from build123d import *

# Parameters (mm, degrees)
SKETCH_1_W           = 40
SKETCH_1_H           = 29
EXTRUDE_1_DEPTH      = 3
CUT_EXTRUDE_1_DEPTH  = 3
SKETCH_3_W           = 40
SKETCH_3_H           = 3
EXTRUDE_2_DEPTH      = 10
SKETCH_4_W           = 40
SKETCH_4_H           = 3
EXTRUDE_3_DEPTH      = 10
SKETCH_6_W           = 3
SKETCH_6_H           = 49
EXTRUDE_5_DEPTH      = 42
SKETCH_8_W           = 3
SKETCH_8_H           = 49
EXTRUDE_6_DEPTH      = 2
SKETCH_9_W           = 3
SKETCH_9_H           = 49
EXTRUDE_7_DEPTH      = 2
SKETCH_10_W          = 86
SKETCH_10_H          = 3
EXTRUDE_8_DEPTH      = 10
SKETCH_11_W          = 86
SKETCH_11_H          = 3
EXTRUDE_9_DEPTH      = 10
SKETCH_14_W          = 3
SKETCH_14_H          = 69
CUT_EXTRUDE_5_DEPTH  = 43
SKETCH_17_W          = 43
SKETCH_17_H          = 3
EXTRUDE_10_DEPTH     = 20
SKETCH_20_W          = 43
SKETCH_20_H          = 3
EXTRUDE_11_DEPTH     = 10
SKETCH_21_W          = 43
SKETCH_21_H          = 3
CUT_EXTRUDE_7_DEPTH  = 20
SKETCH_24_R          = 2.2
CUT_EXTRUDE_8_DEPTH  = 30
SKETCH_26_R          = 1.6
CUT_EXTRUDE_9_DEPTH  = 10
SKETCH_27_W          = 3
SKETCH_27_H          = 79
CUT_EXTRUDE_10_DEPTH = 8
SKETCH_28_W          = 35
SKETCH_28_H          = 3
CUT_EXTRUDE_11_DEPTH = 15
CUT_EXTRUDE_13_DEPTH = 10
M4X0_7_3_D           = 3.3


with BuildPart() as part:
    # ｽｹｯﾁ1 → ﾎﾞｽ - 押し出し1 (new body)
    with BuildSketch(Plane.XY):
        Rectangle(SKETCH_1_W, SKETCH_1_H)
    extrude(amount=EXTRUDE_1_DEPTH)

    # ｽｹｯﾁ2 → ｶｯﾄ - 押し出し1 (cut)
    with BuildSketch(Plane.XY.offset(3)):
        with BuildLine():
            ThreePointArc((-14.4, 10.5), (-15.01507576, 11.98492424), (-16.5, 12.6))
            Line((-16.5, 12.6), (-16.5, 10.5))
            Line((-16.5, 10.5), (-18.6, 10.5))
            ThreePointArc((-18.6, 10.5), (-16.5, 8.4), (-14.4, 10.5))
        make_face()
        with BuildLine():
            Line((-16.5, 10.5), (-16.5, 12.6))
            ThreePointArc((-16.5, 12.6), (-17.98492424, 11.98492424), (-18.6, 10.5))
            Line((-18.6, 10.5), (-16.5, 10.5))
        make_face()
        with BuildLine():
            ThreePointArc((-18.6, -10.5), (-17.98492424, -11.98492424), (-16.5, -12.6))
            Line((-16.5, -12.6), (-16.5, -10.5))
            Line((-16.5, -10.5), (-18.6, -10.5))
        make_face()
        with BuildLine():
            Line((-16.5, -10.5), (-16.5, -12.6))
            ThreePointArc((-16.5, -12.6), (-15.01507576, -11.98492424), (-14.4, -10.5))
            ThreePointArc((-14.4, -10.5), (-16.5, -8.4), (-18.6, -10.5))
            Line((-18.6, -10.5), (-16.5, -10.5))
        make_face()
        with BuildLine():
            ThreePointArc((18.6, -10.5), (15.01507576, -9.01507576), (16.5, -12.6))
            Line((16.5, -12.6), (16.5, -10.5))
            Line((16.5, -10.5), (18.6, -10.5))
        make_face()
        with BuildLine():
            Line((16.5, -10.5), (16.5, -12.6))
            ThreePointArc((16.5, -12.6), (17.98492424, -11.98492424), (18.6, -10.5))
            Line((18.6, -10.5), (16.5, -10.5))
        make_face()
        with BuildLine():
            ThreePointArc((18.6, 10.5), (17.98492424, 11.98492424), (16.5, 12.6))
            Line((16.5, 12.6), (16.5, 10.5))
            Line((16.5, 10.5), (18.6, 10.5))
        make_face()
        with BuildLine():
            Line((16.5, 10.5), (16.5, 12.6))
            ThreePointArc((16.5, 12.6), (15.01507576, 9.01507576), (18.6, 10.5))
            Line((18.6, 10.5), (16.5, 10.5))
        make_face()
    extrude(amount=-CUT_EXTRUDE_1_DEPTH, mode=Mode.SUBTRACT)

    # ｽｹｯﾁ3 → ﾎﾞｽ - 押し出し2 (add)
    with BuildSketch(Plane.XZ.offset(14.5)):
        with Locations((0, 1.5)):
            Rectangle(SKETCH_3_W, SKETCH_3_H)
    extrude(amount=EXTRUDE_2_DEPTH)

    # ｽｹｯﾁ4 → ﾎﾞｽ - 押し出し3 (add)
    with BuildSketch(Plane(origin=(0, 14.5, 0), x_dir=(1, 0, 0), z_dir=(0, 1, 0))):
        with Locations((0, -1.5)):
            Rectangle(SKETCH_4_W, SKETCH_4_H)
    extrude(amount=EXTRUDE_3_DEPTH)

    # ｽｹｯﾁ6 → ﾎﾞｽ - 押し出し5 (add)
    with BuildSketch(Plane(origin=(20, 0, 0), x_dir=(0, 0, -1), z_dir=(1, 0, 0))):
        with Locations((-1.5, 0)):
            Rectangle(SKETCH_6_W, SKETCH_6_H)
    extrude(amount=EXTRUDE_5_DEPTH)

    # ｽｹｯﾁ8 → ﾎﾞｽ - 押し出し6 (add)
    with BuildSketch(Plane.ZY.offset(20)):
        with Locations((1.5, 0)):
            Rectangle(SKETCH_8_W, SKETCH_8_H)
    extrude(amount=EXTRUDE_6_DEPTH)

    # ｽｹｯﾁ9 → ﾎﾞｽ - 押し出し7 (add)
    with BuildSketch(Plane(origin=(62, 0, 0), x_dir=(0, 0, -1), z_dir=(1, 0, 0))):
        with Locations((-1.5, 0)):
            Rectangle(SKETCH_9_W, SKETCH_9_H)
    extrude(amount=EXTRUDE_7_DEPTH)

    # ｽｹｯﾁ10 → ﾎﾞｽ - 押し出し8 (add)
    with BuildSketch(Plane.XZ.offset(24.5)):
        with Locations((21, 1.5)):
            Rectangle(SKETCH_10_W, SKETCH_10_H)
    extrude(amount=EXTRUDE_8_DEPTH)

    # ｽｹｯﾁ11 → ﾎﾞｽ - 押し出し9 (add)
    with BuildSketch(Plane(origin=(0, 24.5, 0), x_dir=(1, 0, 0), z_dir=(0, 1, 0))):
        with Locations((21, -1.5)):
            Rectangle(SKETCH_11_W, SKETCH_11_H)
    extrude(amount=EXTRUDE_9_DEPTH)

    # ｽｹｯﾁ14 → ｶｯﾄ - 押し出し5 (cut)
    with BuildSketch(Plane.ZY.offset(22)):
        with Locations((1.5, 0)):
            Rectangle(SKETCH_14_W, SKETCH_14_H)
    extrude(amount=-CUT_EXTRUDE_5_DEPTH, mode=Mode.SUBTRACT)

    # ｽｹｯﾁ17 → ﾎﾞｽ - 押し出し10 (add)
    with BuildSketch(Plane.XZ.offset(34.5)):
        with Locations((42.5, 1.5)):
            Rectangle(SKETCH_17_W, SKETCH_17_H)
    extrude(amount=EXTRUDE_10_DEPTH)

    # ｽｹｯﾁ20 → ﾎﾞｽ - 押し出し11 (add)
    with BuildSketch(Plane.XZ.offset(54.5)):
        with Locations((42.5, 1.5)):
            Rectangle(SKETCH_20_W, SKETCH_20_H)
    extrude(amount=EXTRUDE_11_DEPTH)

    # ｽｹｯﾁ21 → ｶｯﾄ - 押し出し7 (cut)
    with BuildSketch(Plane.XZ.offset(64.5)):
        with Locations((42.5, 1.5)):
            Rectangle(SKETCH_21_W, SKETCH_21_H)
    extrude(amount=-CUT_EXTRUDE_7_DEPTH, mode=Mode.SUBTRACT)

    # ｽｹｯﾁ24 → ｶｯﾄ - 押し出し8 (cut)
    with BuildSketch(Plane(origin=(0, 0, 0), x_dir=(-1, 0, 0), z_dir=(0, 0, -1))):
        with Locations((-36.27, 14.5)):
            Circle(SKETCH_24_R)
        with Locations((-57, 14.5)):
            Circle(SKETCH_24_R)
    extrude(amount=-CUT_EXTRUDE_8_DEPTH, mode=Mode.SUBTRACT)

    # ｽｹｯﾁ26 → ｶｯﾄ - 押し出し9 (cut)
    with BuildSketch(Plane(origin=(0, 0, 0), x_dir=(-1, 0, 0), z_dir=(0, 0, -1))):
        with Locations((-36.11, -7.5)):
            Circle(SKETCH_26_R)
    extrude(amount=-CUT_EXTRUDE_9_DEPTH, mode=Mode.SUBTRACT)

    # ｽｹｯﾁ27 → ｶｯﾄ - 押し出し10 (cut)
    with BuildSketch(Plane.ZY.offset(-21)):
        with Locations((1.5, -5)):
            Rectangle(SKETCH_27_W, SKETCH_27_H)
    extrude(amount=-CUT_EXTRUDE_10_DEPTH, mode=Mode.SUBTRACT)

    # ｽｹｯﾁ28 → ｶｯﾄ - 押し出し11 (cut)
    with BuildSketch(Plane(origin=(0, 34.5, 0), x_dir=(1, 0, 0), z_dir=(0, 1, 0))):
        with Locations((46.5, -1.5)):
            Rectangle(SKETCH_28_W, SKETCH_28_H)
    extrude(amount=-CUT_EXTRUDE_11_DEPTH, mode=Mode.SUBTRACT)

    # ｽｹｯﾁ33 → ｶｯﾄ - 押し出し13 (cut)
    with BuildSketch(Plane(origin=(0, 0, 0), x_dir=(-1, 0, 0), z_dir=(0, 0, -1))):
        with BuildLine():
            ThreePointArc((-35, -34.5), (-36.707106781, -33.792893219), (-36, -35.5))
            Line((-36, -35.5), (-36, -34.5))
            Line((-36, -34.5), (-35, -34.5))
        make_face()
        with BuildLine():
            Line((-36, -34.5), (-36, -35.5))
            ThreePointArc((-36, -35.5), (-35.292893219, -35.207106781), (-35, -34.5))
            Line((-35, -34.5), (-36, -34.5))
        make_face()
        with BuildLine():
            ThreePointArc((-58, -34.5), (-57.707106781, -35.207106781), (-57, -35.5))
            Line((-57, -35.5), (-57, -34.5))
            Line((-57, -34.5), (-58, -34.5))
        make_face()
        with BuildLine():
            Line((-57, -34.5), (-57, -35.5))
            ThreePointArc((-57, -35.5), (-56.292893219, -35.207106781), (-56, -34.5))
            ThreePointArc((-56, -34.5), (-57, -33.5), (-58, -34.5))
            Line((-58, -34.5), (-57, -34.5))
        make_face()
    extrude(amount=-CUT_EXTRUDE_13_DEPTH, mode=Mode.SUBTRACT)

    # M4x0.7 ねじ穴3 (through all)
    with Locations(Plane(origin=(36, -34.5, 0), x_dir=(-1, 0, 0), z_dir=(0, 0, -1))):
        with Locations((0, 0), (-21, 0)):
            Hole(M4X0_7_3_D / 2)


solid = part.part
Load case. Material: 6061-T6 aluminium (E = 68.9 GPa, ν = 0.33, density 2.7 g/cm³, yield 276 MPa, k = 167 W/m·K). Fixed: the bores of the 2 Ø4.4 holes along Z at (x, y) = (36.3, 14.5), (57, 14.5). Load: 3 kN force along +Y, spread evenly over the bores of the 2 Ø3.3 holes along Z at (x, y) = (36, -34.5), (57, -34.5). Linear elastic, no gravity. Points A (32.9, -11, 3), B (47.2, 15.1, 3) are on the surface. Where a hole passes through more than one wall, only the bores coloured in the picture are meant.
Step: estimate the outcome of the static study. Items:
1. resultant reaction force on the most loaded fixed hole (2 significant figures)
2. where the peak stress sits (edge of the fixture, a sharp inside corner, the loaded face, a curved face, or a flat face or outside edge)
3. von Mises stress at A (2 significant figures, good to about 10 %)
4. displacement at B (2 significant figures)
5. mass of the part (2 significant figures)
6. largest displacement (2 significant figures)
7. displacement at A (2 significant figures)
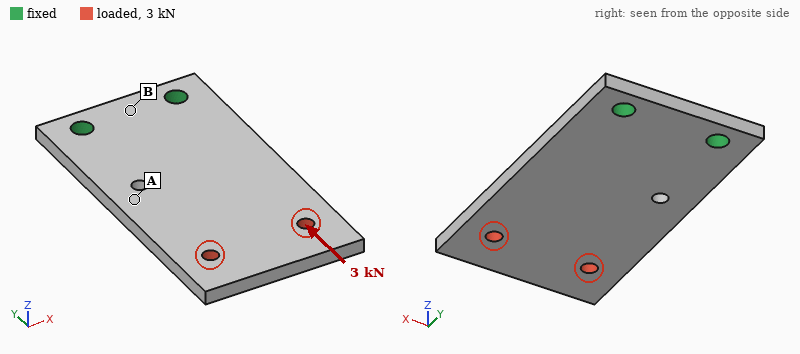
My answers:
1.5 kN
the loaded face
34 MPa
3.8 µm
18 g
25 µm
13 µm
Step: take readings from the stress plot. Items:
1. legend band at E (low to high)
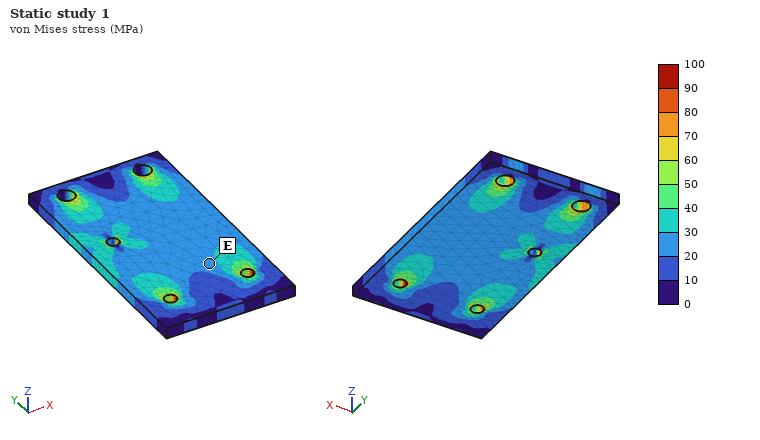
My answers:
20 to 30 MPa
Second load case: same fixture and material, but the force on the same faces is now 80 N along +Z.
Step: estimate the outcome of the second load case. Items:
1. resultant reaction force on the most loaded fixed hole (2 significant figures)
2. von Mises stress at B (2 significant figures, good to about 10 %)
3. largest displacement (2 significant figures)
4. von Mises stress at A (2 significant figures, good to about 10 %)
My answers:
41 N
20 MPa
0.72 mm
37 MPa
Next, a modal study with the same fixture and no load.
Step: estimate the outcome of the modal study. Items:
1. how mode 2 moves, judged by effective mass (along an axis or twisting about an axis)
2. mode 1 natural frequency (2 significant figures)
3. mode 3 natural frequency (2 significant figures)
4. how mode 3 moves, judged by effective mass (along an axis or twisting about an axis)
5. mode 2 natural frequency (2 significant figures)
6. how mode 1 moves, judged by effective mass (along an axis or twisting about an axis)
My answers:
twisting about Y
730 Hz
4500 Hz
along Z
2600 Hz
along Z
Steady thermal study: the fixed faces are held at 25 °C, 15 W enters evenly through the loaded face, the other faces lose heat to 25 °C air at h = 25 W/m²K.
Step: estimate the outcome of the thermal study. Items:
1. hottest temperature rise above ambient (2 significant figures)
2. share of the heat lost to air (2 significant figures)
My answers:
40 K
17 %
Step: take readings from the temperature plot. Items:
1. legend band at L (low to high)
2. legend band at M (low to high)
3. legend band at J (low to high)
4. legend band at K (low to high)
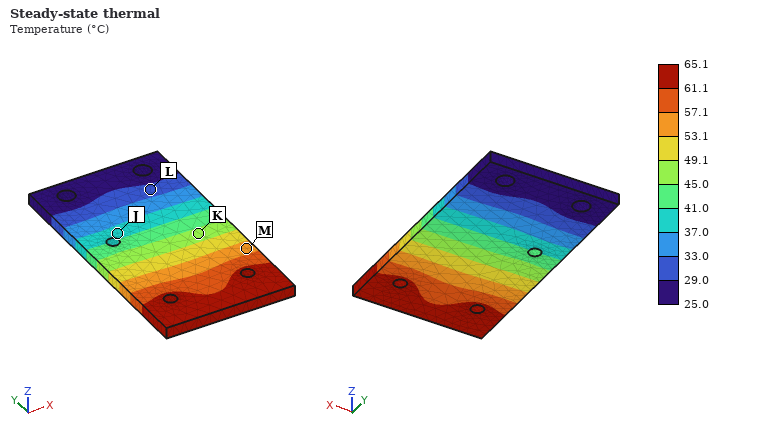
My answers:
29.0 to 33.0 °C
53.1 to 57.1 °C
37.0 to 41.0 °C
45.0 to 49.1 °C
